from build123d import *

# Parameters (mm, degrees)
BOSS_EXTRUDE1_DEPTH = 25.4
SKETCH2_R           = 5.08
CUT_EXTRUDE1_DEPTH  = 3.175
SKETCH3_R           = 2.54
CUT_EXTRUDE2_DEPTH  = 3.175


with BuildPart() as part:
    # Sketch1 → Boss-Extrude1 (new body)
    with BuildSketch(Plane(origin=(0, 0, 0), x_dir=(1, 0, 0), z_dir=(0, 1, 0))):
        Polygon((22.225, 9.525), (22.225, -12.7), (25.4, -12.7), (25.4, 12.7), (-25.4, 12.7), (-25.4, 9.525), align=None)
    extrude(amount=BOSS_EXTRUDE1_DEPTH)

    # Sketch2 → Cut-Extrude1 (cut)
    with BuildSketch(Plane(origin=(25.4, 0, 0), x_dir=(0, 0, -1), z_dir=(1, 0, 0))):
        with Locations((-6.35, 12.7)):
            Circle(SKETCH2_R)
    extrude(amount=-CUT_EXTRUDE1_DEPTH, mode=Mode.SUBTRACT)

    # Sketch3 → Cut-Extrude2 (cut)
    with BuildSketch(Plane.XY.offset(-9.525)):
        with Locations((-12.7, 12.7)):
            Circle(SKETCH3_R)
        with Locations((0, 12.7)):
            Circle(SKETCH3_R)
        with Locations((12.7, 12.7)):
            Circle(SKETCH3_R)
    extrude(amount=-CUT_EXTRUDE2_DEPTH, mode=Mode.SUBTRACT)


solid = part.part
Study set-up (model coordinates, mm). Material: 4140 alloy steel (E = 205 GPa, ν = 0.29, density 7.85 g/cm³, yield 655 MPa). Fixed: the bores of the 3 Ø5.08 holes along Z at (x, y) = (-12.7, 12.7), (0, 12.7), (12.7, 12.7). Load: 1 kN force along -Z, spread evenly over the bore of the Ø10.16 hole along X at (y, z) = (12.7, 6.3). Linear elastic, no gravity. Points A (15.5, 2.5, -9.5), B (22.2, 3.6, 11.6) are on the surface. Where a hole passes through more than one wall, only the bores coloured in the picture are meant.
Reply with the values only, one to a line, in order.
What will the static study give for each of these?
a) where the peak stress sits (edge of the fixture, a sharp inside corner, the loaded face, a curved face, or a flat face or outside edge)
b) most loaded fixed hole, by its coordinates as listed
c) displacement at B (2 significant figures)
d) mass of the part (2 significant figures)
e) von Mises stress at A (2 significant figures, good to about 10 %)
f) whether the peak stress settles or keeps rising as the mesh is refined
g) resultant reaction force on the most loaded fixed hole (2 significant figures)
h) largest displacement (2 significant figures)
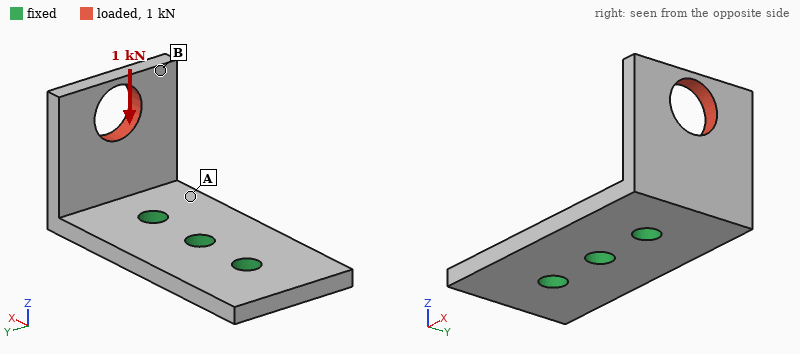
edge of the fixture
(12.7, 12.7)
0.095 mm
43 g
100 MPa
keeps rising
1.2 kN
0.10 mm
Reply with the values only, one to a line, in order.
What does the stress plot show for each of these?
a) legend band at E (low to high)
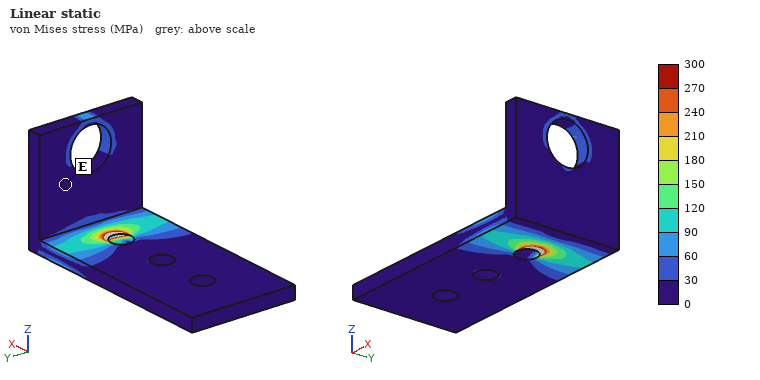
0 to 30 MPa
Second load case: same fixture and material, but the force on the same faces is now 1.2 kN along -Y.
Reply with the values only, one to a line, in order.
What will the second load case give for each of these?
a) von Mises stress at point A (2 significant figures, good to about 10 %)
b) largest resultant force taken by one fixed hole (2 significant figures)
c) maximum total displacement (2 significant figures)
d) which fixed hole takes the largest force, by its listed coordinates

190 MPa
1.6 kN
0.23 mm
(12.7, 12.7)
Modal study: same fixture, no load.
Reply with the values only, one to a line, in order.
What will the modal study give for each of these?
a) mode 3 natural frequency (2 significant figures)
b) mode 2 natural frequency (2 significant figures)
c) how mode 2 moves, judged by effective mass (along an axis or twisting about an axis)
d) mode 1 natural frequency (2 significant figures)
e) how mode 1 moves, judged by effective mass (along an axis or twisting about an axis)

8600 Hz
4400 Hz
along Y
3100 Hz
along X
